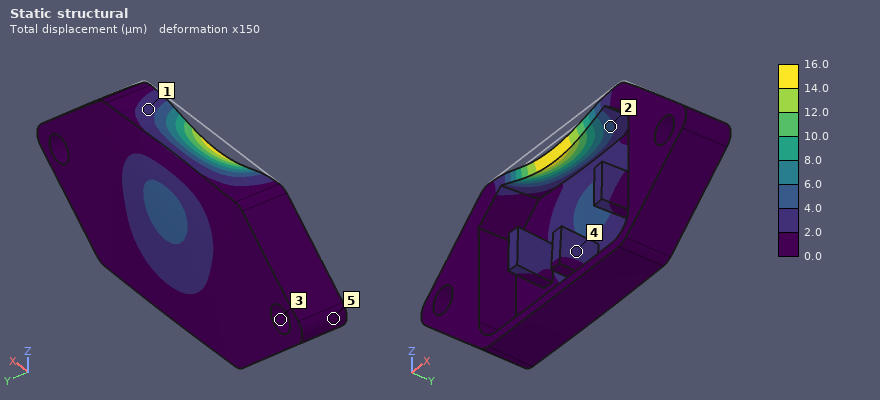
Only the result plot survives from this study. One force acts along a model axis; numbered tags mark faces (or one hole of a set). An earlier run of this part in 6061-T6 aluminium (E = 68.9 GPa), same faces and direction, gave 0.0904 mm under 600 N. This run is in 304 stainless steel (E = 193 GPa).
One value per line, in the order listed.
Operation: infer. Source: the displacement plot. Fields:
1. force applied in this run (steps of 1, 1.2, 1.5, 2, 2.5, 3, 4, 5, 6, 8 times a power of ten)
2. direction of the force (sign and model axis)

300 N
-Z
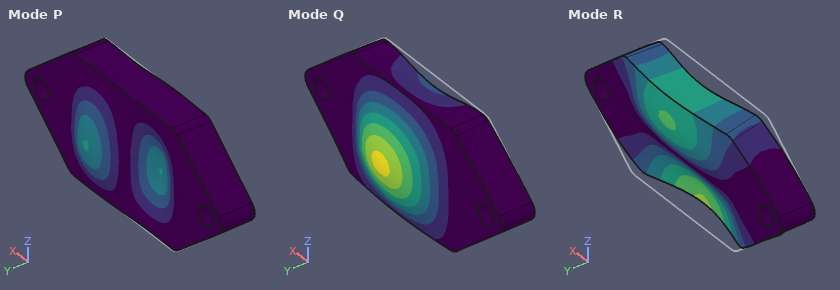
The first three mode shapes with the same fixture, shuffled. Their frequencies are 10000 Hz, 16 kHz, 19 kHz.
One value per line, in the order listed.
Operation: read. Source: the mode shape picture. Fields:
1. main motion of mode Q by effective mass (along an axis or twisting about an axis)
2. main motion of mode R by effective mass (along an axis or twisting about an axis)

along Y
twisting about X
